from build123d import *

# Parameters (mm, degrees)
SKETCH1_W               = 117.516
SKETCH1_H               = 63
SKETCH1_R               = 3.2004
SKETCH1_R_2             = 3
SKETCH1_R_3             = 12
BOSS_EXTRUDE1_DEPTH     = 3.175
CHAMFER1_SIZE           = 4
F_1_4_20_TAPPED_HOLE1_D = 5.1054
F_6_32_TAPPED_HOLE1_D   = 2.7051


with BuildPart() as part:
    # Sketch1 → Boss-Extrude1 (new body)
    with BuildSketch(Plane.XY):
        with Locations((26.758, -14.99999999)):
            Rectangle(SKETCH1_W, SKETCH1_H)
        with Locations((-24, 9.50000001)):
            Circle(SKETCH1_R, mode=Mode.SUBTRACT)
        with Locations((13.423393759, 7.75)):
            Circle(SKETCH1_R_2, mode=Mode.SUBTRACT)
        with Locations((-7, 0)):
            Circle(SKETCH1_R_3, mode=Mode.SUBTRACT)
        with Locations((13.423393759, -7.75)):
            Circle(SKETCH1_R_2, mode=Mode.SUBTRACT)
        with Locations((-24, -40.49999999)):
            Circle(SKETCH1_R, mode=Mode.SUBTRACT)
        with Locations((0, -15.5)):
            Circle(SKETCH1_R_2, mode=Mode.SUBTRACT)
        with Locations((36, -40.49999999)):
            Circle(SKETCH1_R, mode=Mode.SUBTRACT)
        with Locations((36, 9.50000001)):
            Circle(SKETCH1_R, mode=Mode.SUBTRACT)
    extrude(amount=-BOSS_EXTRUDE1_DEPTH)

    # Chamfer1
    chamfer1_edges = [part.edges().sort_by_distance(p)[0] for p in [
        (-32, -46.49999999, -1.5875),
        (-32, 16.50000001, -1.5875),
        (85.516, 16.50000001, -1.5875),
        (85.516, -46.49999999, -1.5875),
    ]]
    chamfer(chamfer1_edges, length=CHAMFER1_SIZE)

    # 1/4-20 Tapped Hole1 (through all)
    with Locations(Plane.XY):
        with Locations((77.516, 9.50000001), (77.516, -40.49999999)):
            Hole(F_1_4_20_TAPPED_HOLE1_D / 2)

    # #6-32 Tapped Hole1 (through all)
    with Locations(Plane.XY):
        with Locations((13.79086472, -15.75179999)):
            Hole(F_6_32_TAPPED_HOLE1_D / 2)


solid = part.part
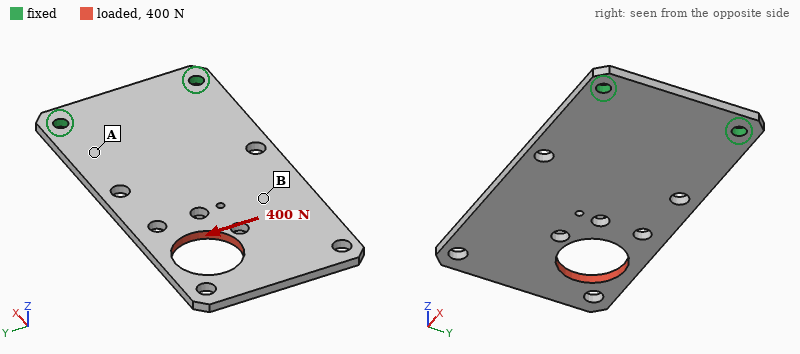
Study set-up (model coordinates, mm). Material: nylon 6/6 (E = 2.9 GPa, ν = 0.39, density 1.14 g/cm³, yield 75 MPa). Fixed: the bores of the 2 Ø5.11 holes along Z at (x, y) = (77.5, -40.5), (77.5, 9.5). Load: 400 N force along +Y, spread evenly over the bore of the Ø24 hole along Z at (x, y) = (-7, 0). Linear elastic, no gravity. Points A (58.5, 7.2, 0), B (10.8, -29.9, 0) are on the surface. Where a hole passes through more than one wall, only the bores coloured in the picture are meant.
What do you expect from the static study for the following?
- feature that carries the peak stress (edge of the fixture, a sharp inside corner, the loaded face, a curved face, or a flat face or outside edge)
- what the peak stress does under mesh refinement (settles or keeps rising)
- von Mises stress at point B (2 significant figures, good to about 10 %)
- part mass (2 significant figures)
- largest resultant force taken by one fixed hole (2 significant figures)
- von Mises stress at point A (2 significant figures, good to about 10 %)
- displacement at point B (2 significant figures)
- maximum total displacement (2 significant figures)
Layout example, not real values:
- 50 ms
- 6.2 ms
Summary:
- edge of the fixture
- keeps rising
- 3.5 MPa
- 24 g
- 690 N
- 9.5 MPa
- 0.49 mm
- 1.0 mm
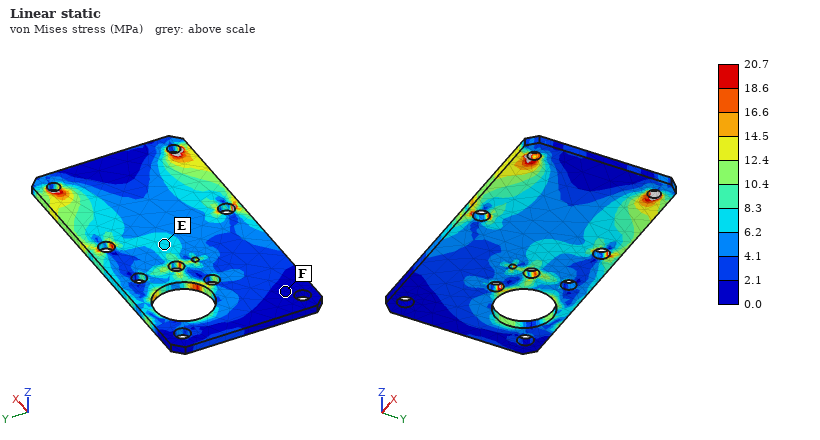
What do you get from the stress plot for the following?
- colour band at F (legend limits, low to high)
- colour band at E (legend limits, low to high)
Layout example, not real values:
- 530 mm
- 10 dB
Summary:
- 0.0 to 2.1 MPa
- 6.2 to 8.3 MPa
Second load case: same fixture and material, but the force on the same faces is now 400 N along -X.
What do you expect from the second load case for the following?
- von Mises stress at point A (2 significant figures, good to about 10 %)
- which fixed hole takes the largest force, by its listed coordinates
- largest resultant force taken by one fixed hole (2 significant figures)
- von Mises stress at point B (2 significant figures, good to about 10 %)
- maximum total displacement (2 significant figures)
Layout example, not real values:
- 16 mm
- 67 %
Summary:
- 4.6 MPa
- (77.5, 9.5)
- 330 N
- 1.2 MPa
- 0.30 mm
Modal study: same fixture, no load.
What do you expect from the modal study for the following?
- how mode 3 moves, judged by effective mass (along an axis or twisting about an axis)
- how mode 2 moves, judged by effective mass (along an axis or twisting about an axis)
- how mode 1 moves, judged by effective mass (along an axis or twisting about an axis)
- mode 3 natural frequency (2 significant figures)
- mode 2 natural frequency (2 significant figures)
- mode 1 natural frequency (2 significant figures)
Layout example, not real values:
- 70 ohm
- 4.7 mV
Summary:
- along Z
- twisting about X
- along Z
- 400 Hz
- 270 Hz
- 72 Hz
